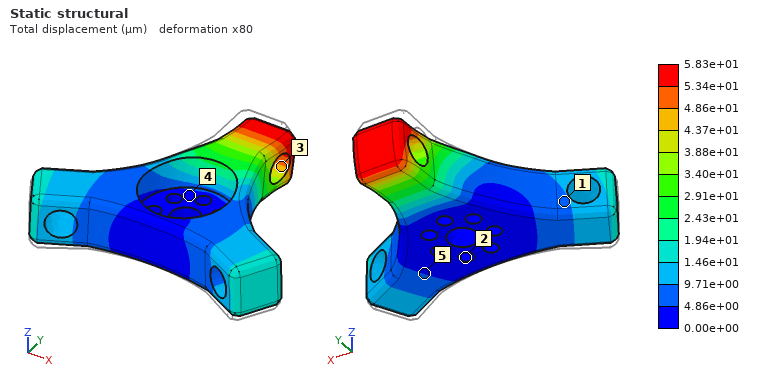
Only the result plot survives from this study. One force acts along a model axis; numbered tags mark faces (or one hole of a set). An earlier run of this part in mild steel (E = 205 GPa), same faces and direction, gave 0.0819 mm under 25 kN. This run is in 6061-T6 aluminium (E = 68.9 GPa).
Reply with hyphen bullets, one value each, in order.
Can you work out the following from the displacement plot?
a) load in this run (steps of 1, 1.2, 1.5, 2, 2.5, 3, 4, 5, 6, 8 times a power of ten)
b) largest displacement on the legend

- 6 kN
- 5.83e+01 µm
